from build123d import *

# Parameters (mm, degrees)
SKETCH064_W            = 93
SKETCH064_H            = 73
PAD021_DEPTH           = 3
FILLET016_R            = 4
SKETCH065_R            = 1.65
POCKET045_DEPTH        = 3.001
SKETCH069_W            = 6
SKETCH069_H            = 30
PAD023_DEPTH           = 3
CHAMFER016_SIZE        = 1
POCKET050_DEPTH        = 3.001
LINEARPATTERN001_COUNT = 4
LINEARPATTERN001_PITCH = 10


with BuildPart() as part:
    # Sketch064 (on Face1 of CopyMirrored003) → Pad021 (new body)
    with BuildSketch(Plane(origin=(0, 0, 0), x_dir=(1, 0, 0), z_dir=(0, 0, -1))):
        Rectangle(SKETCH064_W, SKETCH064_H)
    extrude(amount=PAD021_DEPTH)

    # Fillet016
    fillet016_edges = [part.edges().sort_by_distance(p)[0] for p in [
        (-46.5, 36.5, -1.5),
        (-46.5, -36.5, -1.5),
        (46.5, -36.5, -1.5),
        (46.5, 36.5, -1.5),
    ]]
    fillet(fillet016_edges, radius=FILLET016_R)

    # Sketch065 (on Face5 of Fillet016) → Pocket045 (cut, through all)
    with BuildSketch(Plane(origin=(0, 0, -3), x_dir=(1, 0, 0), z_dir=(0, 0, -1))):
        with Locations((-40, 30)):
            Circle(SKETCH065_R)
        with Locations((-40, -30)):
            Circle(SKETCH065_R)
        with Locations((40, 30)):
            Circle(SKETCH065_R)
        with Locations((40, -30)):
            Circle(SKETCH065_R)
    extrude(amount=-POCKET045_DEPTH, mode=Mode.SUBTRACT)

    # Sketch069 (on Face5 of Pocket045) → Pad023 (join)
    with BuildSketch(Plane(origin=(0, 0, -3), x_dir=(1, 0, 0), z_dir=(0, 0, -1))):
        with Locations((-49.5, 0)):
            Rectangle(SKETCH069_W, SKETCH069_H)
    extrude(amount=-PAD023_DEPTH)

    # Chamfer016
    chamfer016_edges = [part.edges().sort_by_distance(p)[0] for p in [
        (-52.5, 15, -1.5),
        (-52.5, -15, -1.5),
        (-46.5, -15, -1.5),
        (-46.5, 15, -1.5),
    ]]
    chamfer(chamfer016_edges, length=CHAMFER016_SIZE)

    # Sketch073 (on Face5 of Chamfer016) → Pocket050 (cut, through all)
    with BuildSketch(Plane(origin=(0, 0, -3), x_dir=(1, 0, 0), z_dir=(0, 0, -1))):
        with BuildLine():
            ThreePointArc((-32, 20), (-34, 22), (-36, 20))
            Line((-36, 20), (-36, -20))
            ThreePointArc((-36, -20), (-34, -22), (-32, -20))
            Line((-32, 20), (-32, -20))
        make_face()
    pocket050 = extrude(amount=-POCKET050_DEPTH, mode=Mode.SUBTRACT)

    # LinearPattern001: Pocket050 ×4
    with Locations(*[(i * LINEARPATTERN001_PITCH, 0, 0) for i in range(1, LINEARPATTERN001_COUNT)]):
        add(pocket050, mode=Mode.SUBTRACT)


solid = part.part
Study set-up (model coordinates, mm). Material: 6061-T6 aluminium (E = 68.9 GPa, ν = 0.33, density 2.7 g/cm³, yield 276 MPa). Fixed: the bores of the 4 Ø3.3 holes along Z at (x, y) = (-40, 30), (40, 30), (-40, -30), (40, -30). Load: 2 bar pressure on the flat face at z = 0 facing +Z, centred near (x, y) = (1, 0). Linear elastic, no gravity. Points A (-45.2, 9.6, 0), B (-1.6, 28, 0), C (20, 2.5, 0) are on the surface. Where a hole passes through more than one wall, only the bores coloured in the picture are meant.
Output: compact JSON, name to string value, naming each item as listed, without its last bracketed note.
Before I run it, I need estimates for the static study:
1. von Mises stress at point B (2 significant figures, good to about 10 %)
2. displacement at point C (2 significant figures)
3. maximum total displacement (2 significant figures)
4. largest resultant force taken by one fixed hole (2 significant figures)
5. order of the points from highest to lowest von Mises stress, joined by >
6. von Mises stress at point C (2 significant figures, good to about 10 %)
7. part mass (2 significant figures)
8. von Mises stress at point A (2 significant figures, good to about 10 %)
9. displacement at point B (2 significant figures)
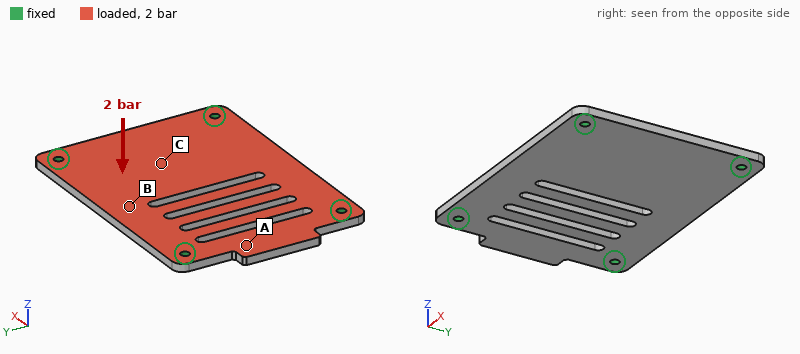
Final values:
{"von Mises stress at point B": "70 MPa", "displacement at point C": "0.20 mm", "maximum total displacement": "0.36 mm", "largest resultant force taken by one fixed hole": "320 N", "order of the points from highest to lowest von Mises stress, joined by >": "B > C > A", "von Mises stress at point C": "25 MPa", "part mass": "50 g", "von Mises stress at point A": "14 MPa", "displacement at point B": "0.25 mm"}
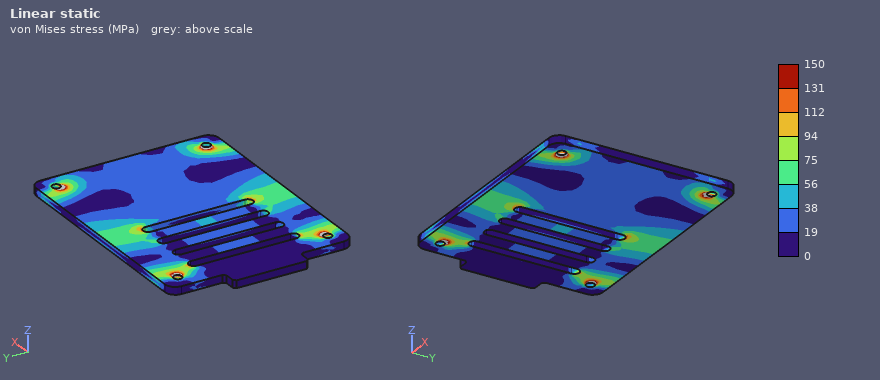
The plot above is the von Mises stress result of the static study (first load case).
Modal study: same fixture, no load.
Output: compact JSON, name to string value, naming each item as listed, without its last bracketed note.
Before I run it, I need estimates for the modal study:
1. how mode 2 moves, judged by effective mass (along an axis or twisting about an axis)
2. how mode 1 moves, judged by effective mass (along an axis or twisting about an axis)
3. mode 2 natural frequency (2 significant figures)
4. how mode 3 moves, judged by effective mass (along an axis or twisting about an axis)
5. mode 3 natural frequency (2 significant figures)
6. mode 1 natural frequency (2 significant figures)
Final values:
{"how mode 2 moves, judged by effective mass": "twisting about X", "how mode 1 moves, judged by effective mass": "along Z", "mode 2 natural frequency": "2800 Hz", "how mode 3 moves, judged by effective mass": "twisting about Y", "mode 3 natural frequency": "3600 Hz", "mode 1 natural frequency": "1700 Hz"}
